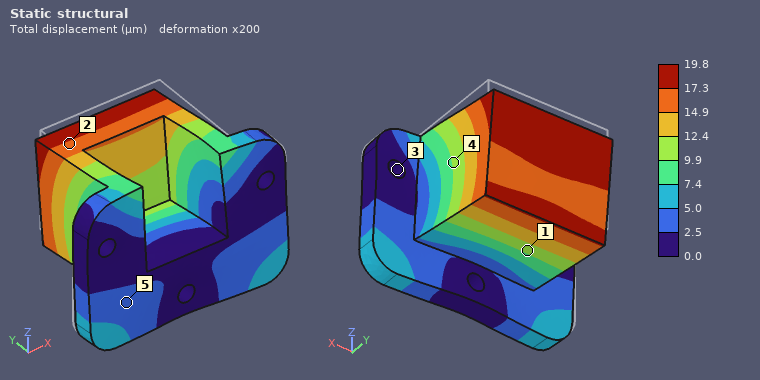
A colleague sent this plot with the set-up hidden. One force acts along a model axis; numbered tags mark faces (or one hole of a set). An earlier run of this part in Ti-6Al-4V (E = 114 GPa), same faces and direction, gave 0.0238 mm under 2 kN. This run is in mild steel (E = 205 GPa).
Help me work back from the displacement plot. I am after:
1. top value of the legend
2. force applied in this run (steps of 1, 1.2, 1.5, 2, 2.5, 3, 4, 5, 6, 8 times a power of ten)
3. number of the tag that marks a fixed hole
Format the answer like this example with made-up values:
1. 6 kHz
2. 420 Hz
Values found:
1. 19.8 µm
2. 3 kN
3. 3
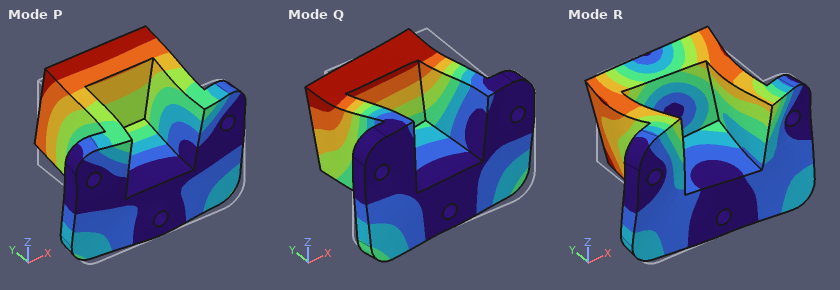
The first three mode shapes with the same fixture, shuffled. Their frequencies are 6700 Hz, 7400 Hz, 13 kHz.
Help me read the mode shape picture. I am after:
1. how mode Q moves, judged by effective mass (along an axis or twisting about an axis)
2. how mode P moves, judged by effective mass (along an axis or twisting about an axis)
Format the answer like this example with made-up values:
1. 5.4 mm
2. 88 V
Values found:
1. along X
2. along Z
